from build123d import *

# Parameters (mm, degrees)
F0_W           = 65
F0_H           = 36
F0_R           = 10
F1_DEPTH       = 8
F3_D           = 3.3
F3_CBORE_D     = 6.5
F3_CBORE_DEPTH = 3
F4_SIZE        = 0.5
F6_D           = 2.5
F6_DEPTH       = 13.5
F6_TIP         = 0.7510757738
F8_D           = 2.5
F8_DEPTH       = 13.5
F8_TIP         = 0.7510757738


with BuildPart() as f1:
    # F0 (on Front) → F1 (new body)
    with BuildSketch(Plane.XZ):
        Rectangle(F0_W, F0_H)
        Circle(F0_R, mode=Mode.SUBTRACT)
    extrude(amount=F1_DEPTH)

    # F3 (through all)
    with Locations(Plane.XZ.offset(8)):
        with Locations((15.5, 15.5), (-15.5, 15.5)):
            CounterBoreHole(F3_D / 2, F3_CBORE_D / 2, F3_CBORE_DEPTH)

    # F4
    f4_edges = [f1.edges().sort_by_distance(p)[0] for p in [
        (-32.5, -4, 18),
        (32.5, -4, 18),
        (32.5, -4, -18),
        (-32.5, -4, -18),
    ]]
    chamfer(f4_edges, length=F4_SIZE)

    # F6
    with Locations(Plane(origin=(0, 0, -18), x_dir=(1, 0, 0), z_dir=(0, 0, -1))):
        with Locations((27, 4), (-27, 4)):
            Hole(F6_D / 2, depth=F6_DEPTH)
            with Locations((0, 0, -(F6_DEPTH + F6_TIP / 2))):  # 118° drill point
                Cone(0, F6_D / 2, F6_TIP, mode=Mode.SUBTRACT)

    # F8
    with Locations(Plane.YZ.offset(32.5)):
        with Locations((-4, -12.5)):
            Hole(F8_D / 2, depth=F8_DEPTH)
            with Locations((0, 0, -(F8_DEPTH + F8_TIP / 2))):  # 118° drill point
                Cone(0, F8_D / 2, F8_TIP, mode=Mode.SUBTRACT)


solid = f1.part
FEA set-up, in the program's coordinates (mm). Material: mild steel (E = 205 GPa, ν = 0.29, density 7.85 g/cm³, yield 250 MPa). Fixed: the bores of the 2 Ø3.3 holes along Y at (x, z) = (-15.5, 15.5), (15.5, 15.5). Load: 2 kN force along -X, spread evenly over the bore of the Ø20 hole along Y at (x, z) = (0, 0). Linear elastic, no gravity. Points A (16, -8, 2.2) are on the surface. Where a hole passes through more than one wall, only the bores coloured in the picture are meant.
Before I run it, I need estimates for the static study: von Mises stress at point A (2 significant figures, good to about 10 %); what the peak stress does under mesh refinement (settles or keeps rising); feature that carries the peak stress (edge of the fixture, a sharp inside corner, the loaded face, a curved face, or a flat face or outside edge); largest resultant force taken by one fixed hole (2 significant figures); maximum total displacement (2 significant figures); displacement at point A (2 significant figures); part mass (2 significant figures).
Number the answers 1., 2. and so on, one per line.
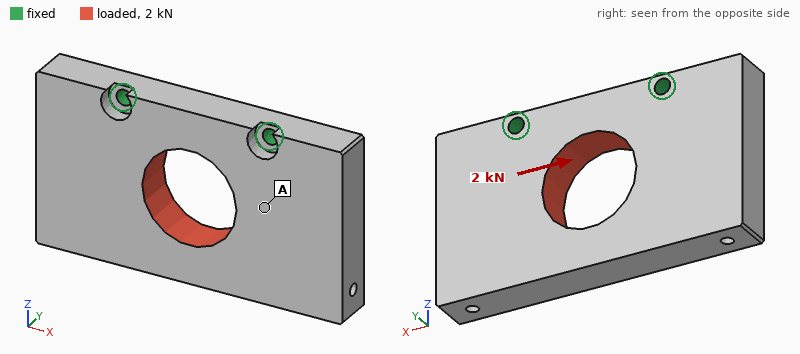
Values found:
1. 10 MPa
2. keeps rising
3. edge of the fixture
4. 1.3 kN
5. 9.4 µm
6. 3.7 µm
7. 120 g
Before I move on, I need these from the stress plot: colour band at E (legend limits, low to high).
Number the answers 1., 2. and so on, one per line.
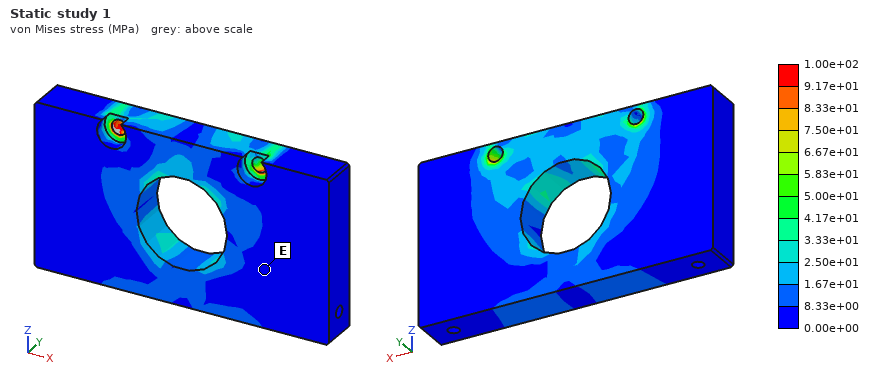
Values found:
1. 0.00e+00 to 8.33e+00 MPa
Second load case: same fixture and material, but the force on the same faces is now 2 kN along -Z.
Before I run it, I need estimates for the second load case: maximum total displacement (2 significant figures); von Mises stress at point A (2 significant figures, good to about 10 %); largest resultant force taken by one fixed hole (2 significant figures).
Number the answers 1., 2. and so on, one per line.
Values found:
1. 6.1 µm
2. 7.5 MPa
3. 1.0 kN
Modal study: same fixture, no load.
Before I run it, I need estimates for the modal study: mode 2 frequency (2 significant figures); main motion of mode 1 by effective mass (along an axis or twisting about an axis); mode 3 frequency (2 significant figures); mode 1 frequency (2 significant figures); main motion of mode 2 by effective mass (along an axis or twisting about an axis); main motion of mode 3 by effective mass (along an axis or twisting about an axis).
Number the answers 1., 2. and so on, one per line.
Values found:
1. 4800 Hz
2. along Y
3. 7500 Hz
4. 2900 Hz
5. twisting about Z
6. along X
